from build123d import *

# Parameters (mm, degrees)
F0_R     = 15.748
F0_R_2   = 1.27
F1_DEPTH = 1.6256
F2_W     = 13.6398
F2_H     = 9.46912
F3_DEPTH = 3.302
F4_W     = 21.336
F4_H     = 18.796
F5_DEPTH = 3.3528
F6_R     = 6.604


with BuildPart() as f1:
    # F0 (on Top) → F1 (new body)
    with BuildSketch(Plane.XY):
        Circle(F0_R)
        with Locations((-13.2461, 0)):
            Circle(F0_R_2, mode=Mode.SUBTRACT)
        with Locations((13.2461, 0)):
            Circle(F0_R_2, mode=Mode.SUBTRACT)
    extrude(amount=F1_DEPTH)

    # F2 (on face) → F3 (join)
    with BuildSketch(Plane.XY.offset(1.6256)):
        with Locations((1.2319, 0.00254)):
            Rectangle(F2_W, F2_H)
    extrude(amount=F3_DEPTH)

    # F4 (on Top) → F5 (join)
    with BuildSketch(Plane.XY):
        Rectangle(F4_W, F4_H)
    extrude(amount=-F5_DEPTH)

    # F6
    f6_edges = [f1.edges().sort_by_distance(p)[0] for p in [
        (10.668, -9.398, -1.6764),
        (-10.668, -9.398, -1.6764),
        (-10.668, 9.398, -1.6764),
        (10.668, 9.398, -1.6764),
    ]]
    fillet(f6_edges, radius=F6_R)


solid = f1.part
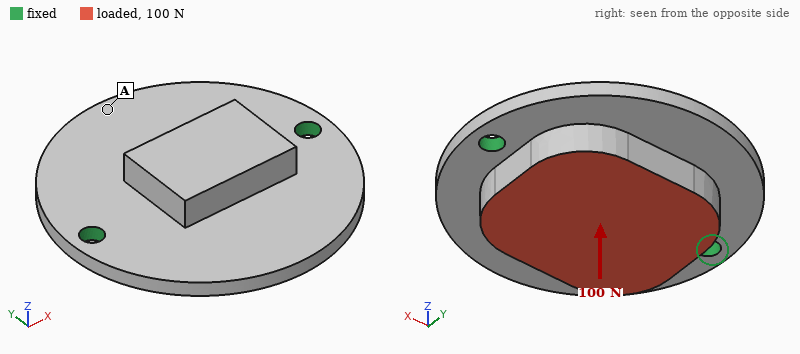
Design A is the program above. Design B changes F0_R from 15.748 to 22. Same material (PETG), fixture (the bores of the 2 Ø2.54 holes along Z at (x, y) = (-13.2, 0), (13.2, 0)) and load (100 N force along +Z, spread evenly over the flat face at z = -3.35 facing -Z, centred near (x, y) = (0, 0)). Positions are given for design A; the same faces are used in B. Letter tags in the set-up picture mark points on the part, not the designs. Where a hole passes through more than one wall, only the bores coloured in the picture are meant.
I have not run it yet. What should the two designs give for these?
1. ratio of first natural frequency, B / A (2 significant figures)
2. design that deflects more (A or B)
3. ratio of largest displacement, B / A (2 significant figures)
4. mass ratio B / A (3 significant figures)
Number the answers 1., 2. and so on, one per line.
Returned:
1. 0.65
2. B
3. 1.2
4. 1.42
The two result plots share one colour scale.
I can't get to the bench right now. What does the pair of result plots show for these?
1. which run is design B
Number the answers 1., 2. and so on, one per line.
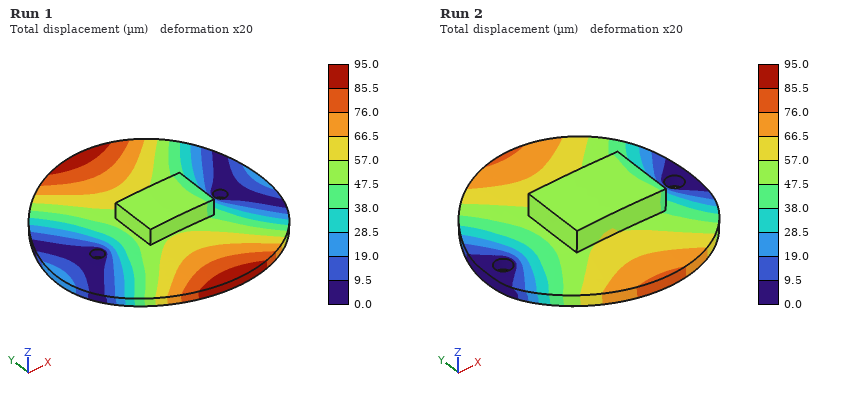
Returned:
1. Run 1
